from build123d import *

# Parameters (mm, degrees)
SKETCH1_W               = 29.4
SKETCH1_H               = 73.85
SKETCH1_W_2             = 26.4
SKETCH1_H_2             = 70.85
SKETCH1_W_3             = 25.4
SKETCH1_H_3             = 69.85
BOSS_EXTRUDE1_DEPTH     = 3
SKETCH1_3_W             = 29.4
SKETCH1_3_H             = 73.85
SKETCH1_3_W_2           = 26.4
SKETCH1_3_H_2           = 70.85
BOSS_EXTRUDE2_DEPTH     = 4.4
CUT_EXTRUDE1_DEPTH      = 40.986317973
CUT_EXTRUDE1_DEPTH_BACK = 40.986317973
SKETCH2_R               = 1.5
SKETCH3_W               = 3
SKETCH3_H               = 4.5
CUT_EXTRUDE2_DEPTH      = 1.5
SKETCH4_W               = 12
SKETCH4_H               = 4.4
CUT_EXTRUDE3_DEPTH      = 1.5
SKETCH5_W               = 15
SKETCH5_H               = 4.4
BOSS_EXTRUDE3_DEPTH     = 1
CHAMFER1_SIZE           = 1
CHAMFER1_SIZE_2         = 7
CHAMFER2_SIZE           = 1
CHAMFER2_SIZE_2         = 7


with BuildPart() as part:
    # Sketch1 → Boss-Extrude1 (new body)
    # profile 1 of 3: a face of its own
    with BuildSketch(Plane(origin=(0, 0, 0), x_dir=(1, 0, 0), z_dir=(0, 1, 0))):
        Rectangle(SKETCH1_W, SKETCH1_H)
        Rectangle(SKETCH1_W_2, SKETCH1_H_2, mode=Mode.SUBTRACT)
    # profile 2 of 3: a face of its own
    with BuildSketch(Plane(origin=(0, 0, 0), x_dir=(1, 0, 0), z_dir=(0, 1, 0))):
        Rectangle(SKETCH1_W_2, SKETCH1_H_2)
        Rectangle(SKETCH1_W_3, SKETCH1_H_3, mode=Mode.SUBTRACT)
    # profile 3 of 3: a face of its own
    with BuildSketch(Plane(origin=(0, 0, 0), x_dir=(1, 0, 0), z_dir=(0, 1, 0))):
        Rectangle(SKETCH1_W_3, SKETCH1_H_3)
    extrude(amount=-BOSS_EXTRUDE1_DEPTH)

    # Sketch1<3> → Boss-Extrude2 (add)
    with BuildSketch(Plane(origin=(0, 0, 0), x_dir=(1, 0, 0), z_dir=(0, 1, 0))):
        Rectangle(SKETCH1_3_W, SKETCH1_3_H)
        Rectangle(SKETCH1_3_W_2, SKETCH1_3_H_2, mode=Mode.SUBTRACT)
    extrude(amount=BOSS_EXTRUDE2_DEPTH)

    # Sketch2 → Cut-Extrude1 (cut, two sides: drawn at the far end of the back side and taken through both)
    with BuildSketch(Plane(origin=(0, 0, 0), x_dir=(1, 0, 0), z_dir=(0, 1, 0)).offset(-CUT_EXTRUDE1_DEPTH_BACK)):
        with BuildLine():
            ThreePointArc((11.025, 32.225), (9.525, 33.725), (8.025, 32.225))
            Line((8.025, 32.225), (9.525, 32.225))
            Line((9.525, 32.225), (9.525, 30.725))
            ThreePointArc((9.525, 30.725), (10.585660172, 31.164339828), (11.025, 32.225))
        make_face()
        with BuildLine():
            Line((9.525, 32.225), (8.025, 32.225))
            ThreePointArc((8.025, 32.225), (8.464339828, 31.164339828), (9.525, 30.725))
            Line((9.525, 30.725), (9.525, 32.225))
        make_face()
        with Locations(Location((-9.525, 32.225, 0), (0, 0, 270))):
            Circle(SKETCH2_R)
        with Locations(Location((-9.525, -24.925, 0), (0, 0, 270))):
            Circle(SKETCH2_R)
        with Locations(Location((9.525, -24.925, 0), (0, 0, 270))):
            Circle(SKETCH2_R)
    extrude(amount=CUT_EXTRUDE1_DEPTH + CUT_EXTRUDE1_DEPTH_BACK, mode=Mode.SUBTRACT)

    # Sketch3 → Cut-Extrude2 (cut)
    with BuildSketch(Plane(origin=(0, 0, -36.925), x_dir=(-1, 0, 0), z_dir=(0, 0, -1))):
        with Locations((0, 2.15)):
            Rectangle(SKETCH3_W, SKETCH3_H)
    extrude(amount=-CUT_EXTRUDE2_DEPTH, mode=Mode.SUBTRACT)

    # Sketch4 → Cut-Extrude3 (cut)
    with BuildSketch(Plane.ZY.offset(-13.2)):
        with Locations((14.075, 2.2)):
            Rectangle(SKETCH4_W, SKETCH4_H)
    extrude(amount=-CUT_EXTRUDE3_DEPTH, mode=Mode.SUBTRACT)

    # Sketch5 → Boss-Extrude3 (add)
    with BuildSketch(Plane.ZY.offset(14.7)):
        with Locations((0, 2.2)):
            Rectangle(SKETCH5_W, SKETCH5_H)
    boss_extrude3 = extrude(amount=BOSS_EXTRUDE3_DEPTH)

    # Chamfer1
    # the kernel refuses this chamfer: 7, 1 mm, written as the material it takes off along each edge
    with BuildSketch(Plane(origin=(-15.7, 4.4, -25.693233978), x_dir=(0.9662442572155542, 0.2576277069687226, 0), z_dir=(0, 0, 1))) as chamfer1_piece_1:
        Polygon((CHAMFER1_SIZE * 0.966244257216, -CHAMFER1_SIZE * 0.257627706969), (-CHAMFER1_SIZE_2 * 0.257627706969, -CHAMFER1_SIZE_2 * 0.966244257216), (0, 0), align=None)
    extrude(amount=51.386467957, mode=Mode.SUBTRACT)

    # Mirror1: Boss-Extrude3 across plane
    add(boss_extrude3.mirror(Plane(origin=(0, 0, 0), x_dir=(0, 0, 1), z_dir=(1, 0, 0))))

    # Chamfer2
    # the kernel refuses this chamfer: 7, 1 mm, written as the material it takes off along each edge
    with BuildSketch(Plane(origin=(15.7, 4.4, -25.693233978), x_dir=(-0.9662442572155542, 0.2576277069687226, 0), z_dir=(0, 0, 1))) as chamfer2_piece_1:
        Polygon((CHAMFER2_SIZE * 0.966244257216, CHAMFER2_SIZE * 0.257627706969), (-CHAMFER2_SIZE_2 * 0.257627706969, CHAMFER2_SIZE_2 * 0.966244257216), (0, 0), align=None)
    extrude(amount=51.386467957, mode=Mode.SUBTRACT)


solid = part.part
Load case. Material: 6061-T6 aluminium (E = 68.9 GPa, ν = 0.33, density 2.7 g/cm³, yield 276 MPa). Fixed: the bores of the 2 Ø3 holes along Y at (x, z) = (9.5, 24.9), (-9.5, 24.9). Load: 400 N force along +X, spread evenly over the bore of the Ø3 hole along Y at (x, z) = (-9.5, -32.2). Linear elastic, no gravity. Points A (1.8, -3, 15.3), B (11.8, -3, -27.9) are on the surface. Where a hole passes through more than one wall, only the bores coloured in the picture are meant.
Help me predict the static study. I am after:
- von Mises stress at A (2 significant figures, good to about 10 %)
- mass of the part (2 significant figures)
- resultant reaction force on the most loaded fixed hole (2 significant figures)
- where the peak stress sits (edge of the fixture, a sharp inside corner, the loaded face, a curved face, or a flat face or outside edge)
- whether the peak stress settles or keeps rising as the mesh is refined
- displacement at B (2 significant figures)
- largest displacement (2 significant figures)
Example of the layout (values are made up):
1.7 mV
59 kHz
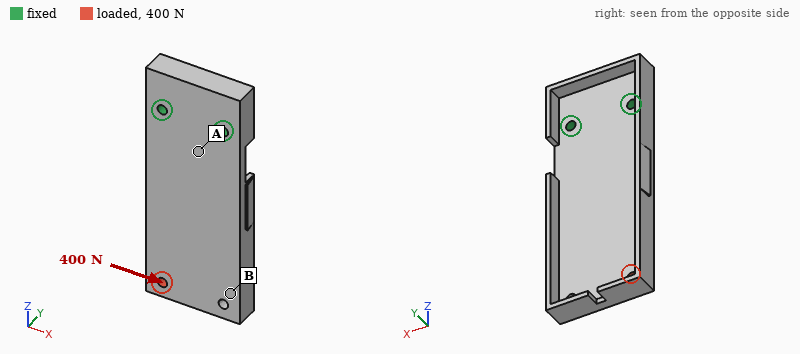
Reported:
14 MPa
21 g
1.1 kN
edge of the fixture
keeps rising
0.079 mm
0.11 mm
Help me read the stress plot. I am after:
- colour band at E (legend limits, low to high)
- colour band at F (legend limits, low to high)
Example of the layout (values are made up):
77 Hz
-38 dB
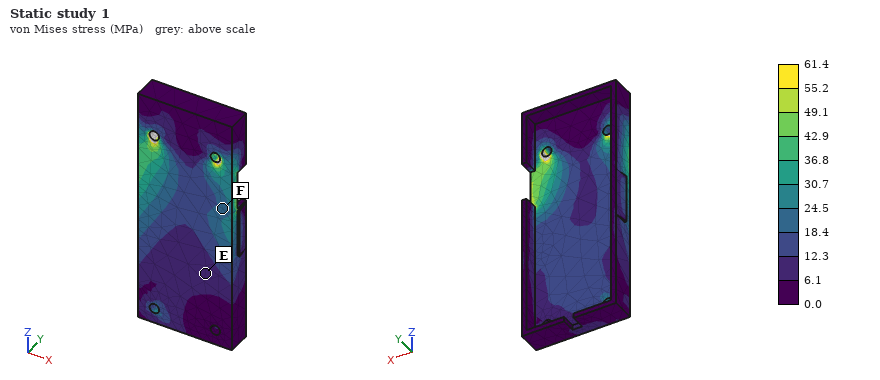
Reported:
6.1 to 12.3 MPa
18.4 to 24.5 MPa
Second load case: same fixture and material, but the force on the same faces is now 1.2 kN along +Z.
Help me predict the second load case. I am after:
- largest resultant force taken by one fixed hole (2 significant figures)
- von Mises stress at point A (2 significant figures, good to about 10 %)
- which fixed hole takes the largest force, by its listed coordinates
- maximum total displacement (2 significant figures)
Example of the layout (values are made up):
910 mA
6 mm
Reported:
1.2 kN
14 MPa
(-9.5, 24.9)
0.12 mm
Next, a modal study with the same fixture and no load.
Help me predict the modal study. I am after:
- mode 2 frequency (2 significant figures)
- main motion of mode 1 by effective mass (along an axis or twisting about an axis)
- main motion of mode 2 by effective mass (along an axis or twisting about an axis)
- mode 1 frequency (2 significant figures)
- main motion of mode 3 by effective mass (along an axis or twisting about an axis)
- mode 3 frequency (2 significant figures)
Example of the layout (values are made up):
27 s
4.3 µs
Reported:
2500 Hz
along Y
twisting about Z
780 Hz
along X
4900 Hz
